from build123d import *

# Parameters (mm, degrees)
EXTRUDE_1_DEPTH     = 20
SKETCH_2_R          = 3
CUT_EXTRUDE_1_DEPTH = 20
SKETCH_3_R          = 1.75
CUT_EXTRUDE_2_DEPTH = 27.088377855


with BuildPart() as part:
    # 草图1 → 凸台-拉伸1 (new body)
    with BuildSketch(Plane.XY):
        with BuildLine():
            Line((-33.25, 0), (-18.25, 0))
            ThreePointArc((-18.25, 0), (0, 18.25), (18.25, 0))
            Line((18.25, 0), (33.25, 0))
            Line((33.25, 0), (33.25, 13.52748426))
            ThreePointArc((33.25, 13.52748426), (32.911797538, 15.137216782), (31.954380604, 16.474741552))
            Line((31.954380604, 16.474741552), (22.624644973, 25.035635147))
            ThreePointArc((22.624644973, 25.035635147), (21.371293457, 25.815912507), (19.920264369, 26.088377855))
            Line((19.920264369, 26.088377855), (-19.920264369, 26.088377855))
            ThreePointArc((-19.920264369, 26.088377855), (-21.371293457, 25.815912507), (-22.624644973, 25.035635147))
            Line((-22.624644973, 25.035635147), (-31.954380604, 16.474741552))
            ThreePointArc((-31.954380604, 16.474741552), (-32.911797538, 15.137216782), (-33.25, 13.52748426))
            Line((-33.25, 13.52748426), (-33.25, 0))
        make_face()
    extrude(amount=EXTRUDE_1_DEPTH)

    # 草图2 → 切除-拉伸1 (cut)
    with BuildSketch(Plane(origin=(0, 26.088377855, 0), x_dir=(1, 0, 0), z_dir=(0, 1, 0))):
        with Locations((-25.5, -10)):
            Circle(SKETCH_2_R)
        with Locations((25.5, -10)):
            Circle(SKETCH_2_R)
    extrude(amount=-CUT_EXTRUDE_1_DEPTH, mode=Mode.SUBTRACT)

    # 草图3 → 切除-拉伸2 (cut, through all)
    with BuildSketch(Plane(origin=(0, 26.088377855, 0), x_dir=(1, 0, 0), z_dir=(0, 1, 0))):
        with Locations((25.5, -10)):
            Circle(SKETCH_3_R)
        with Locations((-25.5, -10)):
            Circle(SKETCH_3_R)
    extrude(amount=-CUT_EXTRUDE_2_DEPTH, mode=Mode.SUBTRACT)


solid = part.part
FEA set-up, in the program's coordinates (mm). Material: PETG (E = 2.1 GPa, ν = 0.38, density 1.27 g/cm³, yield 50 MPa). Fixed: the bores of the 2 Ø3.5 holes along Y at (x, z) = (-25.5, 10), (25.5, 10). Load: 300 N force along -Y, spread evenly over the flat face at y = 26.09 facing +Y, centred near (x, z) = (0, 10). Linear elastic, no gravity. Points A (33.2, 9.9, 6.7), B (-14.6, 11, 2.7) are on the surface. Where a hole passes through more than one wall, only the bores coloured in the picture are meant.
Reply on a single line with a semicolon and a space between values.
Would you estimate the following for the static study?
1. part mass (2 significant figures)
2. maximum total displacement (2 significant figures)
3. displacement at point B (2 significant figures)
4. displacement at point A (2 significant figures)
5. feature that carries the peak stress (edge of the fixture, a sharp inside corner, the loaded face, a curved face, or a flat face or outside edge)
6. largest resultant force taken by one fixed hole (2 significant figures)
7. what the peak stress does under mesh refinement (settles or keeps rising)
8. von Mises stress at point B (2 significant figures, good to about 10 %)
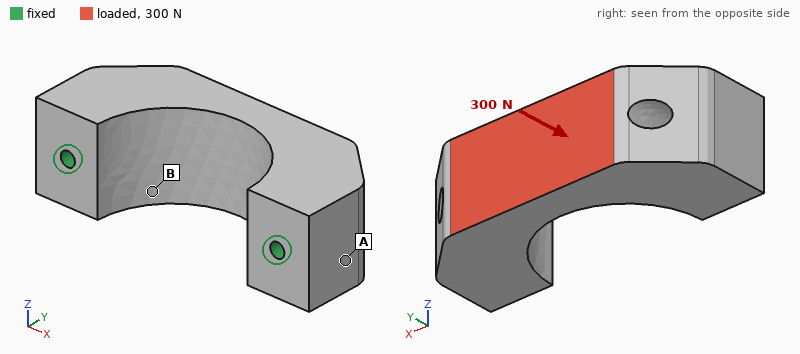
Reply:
26 g; 33 µm; 17 µm; 5.5 µm; edge of the fixture; 180 N; keeps rising; 1.6 MPa
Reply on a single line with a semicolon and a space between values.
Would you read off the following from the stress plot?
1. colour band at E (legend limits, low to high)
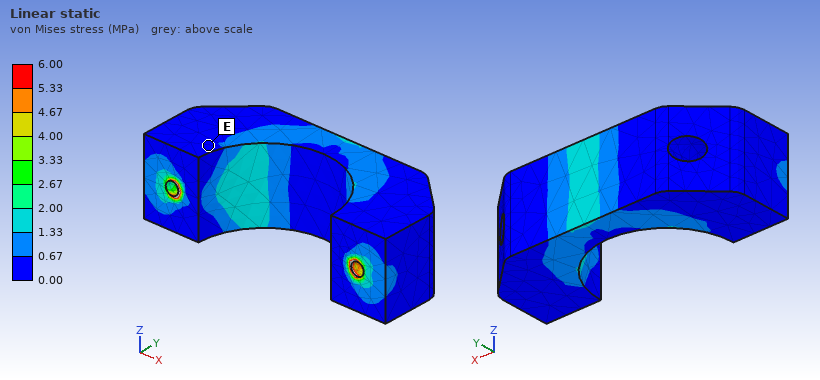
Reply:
0.00 to 0.67 MPa
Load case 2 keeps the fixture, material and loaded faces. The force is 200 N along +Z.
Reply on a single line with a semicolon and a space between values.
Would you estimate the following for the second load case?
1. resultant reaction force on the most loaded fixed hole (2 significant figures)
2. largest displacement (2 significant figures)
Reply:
100 N; 0.30 mm
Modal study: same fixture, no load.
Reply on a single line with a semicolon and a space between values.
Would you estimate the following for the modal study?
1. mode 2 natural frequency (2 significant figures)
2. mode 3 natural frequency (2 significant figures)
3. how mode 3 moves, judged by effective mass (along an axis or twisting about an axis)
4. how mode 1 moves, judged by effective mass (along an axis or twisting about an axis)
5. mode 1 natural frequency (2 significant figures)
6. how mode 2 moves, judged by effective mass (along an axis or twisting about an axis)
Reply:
2800 Hz; 3200 Hz; along X; along Z; 1400 Hz; twisting about Y
